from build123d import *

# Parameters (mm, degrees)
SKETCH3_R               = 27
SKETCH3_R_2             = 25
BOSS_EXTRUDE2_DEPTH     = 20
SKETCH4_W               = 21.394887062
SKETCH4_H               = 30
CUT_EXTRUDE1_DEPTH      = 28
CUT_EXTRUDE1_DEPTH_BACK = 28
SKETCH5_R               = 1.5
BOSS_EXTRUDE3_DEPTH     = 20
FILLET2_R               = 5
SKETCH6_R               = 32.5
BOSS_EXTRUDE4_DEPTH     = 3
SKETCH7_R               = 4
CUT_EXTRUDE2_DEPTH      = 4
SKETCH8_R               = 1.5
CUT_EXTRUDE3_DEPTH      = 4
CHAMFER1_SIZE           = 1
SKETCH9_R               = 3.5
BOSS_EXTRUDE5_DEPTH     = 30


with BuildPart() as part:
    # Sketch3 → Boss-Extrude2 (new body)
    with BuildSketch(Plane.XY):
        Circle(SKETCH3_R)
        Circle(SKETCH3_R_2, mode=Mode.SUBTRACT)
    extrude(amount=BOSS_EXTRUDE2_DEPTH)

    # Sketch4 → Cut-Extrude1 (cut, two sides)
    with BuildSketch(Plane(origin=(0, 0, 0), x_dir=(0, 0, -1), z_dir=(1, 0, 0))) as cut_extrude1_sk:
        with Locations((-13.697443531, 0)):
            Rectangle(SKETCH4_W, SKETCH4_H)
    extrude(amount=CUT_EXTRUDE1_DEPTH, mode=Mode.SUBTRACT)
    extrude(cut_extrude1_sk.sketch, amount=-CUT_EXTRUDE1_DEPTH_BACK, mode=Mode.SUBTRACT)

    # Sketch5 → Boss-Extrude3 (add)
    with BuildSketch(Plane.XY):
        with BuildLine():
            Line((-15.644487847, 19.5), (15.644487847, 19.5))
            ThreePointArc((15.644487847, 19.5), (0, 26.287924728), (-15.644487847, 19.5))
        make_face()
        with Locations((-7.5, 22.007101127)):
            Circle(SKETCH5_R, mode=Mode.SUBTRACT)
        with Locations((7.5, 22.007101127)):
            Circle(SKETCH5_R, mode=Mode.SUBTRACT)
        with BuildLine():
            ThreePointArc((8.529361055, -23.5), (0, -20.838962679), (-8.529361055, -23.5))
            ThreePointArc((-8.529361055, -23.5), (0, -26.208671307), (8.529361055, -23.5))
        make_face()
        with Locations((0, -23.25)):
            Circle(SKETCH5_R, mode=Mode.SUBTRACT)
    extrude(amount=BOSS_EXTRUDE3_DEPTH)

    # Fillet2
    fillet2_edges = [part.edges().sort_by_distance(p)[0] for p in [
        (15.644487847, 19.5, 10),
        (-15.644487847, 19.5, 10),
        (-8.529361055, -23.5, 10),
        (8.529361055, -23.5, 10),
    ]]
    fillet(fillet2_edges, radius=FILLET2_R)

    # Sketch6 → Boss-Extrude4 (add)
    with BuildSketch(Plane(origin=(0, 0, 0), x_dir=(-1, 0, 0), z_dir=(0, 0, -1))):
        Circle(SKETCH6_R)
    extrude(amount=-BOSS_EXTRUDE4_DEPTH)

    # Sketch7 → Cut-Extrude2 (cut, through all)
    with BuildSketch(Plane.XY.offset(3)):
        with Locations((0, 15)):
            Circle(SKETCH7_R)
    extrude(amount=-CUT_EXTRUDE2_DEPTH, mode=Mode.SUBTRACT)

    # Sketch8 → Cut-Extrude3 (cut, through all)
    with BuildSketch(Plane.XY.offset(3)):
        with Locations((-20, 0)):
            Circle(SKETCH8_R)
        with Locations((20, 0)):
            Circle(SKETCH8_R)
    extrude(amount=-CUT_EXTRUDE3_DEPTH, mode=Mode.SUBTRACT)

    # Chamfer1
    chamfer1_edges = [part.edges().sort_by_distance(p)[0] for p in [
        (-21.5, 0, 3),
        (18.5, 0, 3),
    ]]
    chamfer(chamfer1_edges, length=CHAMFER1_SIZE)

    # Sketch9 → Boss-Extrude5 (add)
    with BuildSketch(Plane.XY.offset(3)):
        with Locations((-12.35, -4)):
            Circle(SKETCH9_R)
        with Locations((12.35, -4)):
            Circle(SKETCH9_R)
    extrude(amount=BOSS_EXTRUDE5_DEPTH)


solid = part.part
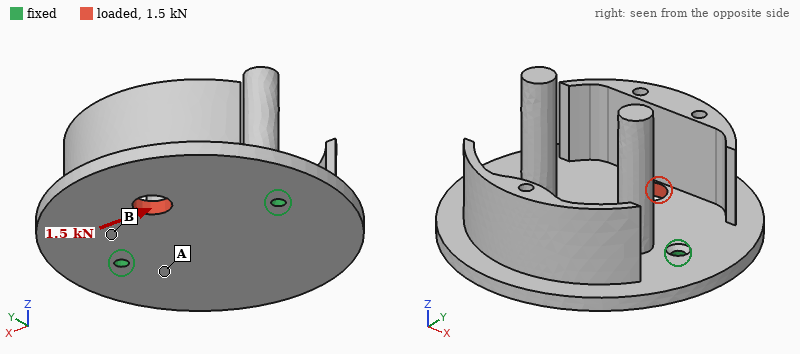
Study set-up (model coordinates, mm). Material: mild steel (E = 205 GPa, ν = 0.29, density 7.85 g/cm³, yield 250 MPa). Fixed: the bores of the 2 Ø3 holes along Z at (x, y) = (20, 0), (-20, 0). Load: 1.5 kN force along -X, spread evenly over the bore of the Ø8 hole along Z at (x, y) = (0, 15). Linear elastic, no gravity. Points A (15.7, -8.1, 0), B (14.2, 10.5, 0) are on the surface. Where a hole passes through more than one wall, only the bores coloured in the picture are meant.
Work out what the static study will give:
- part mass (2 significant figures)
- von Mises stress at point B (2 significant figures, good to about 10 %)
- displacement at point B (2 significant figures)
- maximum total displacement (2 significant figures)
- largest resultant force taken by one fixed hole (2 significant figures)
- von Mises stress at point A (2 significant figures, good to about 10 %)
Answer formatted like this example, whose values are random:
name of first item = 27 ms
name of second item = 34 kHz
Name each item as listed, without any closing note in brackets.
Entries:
part mass = 140 g
von Mises stress at point B = 18 MPa
displacement at point B = 2.0 µm
maximum total displacement = 3.8 µm
largest resultant force taken by one fixed hole = 930 N
von Mises stress at point A = 5.4 MPa
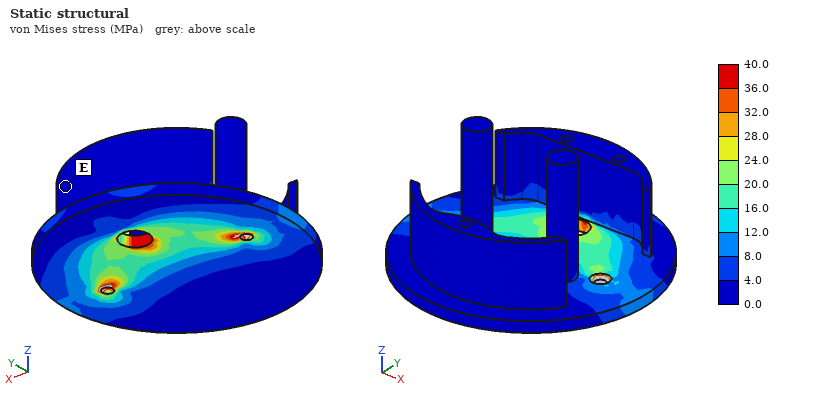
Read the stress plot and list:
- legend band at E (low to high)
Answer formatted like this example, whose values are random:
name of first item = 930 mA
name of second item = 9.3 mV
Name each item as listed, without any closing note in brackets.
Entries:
legend band at E = 0.0 to 4.0 MPa
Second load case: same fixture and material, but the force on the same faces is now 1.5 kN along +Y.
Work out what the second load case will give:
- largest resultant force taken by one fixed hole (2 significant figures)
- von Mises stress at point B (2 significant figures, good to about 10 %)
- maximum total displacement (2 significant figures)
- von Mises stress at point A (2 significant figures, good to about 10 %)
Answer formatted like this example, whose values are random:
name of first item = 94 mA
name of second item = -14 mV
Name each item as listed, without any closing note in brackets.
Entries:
largest resultant force taken by one fixed hole = 760 N
von Mises stress at point B = 12 MPa
maximum total displacement = 4.9 µm
von Mises stress at point A = 8.2 MPa
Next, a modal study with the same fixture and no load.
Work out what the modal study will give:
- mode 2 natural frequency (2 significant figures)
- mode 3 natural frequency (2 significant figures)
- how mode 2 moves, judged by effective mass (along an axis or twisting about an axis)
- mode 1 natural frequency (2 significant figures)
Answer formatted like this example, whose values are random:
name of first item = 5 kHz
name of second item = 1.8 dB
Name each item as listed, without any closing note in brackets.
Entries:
mode 2 natural frequency = 1800 Hz
mode 3 natural frequency = 3500 Hz
how mode 2 moves, judged by effective mass = along Z
mode 1 natural frequency = 1200 Hz
